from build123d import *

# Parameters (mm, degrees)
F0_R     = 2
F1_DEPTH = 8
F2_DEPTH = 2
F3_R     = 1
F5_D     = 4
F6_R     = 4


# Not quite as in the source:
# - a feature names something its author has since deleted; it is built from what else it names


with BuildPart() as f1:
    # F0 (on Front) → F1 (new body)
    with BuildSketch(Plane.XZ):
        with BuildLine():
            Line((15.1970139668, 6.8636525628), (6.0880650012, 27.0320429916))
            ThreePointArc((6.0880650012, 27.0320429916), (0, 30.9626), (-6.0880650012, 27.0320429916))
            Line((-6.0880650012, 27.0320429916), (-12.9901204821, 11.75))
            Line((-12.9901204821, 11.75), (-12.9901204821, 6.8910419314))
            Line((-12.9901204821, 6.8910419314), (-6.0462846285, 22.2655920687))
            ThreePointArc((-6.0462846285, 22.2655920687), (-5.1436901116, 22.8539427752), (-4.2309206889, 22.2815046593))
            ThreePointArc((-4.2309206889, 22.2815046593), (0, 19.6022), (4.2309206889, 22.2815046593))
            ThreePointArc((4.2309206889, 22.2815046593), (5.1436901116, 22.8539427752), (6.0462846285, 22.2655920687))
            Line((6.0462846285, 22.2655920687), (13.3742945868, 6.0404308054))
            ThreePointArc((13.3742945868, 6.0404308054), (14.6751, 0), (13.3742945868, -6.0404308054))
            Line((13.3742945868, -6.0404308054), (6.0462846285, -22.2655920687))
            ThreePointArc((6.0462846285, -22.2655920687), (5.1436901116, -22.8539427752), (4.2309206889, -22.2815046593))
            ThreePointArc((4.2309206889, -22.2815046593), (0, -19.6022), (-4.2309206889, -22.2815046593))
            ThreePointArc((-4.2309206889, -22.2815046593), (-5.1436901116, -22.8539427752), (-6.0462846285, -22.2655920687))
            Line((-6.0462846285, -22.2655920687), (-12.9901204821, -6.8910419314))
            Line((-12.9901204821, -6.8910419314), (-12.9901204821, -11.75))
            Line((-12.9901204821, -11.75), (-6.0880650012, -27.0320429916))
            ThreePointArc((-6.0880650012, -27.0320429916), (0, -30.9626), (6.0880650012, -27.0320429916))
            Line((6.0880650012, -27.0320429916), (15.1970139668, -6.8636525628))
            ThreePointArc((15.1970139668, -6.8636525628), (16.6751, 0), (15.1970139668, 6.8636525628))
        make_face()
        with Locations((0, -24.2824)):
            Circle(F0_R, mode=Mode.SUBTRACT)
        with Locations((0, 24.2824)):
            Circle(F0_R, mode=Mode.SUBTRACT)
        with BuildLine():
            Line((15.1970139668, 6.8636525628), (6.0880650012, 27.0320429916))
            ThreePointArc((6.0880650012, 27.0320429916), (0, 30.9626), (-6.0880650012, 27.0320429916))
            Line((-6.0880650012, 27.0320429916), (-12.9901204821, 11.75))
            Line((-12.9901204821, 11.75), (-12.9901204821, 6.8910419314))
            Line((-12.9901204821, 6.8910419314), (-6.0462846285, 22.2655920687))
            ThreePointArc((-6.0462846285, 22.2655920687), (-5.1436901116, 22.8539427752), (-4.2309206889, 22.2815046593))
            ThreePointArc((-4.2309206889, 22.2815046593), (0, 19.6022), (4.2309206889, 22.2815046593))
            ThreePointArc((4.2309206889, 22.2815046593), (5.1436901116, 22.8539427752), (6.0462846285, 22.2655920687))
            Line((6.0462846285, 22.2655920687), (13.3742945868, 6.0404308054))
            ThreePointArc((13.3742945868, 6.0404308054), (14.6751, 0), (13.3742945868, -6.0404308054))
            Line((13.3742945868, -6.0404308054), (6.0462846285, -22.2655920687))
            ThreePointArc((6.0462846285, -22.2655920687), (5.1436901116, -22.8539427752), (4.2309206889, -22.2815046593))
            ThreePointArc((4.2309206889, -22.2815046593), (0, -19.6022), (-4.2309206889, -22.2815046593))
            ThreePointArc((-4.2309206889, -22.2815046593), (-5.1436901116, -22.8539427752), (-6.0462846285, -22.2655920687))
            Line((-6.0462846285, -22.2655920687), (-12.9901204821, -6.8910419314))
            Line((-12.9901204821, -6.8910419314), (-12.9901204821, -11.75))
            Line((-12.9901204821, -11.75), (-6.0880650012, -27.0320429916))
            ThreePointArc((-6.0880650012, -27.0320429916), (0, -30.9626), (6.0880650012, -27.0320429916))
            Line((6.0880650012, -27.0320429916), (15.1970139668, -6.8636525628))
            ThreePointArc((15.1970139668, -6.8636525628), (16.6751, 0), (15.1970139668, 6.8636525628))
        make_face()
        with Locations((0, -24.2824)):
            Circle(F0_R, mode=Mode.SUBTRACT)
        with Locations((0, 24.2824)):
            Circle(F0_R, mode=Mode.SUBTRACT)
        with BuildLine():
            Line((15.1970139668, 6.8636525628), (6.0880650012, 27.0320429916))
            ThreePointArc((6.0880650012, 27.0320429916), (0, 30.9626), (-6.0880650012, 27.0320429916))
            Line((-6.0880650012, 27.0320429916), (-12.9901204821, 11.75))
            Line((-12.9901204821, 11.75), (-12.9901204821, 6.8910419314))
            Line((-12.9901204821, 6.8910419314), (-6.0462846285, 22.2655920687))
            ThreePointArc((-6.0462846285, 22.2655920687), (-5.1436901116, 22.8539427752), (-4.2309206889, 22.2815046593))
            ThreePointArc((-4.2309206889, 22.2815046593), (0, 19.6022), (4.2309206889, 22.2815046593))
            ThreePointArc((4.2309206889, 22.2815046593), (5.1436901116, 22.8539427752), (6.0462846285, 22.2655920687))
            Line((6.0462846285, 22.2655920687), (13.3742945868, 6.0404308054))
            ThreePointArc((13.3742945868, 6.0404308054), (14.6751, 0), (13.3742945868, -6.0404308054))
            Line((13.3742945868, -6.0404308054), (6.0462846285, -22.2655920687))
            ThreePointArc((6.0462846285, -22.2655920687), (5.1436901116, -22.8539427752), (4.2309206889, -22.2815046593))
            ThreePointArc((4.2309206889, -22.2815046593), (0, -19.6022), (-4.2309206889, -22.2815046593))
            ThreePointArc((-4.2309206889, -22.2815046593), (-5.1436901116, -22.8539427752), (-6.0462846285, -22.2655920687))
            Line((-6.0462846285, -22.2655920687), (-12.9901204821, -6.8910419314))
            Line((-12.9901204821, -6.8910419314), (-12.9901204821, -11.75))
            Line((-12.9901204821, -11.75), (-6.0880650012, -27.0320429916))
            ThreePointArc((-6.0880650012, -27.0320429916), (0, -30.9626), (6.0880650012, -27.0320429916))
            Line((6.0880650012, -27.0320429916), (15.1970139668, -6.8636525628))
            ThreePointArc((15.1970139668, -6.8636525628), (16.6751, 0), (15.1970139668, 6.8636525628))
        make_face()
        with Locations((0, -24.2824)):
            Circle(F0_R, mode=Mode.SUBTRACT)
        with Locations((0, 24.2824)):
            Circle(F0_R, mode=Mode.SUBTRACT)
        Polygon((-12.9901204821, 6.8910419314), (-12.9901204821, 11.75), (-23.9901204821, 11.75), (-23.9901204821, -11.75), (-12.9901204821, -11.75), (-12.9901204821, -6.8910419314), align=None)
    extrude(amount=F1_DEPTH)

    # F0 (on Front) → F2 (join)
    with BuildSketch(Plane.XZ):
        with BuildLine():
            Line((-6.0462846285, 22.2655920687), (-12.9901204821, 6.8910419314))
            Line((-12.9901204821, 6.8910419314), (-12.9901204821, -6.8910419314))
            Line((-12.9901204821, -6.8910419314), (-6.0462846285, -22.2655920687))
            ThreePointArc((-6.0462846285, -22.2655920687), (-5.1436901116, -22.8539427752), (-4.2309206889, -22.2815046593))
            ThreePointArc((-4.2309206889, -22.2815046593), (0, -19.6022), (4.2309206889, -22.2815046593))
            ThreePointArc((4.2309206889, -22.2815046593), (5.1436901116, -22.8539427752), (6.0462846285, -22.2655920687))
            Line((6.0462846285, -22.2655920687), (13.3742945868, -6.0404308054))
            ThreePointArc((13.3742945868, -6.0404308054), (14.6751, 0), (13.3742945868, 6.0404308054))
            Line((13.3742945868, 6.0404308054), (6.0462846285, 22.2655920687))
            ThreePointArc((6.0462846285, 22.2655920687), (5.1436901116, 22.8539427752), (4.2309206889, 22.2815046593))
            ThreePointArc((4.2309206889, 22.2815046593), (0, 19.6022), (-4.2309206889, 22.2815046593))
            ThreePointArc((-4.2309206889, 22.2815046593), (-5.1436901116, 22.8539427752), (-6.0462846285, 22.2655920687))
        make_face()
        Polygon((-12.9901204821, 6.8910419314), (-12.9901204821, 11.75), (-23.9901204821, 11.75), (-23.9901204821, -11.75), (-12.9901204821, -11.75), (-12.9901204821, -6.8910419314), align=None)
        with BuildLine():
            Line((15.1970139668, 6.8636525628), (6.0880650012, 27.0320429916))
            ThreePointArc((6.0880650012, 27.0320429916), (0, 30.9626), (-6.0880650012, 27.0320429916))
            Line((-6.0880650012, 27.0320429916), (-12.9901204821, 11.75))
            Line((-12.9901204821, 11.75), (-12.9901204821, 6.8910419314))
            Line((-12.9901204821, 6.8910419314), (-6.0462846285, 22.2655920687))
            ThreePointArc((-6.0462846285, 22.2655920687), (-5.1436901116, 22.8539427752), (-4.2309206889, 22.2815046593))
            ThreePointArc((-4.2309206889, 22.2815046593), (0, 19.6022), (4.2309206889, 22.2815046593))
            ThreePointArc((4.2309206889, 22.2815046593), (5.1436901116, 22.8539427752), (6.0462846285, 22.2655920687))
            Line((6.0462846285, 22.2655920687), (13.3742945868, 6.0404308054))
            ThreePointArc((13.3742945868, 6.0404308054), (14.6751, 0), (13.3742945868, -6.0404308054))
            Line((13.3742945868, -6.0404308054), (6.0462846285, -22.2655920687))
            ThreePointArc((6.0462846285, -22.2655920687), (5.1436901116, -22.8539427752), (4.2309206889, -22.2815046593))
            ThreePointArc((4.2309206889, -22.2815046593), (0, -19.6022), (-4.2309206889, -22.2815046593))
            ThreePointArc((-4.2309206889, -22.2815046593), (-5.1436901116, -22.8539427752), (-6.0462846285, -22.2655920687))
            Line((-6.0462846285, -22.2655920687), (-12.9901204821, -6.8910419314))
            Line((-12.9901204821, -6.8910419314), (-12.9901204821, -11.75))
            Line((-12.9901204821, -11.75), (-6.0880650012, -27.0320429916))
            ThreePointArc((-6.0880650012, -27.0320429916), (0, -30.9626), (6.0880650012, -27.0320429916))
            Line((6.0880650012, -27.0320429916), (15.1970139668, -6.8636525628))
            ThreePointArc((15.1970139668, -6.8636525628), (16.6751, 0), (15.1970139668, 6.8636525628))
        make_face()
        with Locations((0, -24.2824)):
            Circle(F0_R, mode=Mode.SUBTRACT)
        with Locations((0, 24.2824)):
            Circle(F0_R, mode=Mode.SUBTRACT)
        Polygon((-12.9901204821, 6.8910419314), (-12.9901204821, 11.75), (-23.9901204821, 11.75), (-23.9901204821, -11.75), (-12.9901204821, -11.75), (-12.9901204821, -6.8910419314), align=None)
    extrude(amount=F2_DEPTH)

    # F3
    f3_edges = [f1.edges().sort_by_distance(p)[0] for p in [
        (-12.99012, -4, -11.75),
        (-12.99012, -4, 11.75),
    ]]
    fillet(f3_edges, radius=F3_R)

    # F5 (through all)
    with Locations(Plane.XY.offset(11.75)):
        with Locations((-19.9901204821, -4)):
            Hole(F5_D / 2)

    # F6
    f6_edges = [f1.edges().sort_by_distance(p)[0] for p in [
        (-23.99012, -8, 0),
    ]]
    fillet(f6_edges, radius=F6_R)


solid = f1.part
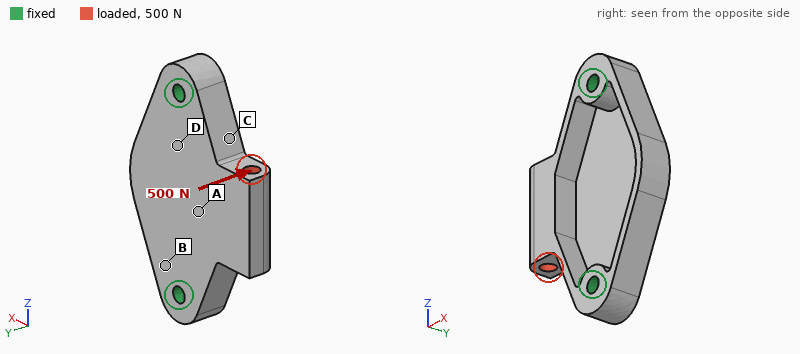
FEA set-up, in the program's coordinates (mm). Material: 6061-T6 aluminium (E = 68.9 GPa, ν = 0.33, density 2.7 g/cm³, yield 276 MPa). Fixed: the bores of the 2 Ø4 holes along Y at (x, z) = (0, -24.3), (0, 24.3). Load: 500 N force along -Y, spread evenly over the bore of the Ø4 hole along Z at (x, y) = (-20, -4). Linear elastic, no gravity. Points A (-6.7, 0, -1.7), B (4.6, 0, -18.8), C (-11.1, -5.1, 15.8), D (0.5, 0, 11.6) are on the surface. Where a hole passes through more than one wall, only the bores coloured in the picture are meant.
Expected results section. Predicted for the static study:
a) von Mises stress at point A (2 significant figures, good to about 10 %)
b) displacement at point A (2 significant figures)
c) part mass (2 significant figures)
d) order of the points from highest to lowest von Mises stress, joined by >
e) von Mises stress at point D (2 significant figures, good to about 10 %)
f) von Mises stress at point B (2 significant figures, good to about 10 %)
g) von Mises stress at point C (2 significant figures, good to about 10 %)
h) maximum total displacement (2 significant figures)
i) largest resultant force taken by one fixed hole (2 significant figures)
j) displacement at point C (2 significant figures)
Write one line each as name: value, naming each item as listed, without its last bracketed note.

von Mises stress at point A: 54 MPa
displacement at point A: 0.034 mm
part mass: 17 g
order of the points from highest to lowest von Mises stress, joined by >: C > A > D > B
von Mises stress at point D: 28 MPa
von Mises stress at point B: 15 MPa
von Mises stress at point C: 140 MPa
maximum total displacement: 0.22 mm
largest resultant force taken by one fixed hole: 580 N
displacement at point C: 0.057 mm
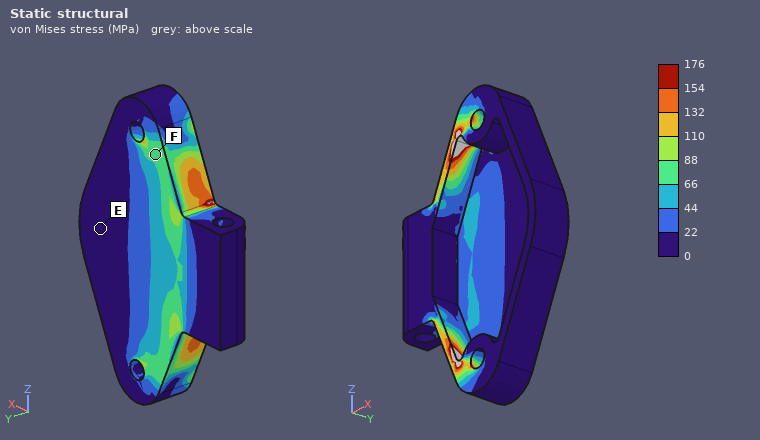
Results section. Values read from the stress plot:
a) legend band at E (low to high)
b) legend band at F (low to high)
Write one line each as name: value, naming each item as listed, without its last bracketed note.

legend band at E: 0 to 22 MPa
legend band at F: 66 to 88 MPa
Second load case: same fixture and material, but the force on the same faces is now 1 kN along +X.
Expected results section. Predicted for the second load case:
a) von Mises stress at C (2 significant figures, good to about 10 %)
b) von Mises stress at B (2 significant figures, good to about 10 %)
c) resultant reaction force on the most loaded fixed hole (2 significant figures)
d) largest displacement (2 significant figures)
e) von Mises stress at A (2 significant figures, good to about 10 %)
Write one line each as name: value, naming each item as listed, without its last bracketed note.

von Mises stress at C: 64 MPa
von Mises stress at B: 16 MPa
resultant reaction force on the most loaded fixed hole: 630 N
largest displacement: 85 µm
von Mises stress at A: 19 MPa
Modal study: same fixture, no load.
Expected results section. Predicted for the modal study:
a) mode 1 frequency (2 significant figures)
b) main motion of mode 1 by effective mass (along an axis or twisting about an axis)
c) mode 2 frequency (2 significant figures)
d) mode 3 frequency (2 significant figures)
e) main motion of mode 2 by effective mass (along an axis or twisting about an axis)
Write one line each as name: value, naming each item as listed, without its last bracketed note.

mode 1 frequency: 4200 Hz
main motion of mode 1 by effective mass: along Y
mode 2 frequency: 8900 Hz
mode 3 frequency: 12 kHz
main motion of mode 2 by effective mass: along Y
